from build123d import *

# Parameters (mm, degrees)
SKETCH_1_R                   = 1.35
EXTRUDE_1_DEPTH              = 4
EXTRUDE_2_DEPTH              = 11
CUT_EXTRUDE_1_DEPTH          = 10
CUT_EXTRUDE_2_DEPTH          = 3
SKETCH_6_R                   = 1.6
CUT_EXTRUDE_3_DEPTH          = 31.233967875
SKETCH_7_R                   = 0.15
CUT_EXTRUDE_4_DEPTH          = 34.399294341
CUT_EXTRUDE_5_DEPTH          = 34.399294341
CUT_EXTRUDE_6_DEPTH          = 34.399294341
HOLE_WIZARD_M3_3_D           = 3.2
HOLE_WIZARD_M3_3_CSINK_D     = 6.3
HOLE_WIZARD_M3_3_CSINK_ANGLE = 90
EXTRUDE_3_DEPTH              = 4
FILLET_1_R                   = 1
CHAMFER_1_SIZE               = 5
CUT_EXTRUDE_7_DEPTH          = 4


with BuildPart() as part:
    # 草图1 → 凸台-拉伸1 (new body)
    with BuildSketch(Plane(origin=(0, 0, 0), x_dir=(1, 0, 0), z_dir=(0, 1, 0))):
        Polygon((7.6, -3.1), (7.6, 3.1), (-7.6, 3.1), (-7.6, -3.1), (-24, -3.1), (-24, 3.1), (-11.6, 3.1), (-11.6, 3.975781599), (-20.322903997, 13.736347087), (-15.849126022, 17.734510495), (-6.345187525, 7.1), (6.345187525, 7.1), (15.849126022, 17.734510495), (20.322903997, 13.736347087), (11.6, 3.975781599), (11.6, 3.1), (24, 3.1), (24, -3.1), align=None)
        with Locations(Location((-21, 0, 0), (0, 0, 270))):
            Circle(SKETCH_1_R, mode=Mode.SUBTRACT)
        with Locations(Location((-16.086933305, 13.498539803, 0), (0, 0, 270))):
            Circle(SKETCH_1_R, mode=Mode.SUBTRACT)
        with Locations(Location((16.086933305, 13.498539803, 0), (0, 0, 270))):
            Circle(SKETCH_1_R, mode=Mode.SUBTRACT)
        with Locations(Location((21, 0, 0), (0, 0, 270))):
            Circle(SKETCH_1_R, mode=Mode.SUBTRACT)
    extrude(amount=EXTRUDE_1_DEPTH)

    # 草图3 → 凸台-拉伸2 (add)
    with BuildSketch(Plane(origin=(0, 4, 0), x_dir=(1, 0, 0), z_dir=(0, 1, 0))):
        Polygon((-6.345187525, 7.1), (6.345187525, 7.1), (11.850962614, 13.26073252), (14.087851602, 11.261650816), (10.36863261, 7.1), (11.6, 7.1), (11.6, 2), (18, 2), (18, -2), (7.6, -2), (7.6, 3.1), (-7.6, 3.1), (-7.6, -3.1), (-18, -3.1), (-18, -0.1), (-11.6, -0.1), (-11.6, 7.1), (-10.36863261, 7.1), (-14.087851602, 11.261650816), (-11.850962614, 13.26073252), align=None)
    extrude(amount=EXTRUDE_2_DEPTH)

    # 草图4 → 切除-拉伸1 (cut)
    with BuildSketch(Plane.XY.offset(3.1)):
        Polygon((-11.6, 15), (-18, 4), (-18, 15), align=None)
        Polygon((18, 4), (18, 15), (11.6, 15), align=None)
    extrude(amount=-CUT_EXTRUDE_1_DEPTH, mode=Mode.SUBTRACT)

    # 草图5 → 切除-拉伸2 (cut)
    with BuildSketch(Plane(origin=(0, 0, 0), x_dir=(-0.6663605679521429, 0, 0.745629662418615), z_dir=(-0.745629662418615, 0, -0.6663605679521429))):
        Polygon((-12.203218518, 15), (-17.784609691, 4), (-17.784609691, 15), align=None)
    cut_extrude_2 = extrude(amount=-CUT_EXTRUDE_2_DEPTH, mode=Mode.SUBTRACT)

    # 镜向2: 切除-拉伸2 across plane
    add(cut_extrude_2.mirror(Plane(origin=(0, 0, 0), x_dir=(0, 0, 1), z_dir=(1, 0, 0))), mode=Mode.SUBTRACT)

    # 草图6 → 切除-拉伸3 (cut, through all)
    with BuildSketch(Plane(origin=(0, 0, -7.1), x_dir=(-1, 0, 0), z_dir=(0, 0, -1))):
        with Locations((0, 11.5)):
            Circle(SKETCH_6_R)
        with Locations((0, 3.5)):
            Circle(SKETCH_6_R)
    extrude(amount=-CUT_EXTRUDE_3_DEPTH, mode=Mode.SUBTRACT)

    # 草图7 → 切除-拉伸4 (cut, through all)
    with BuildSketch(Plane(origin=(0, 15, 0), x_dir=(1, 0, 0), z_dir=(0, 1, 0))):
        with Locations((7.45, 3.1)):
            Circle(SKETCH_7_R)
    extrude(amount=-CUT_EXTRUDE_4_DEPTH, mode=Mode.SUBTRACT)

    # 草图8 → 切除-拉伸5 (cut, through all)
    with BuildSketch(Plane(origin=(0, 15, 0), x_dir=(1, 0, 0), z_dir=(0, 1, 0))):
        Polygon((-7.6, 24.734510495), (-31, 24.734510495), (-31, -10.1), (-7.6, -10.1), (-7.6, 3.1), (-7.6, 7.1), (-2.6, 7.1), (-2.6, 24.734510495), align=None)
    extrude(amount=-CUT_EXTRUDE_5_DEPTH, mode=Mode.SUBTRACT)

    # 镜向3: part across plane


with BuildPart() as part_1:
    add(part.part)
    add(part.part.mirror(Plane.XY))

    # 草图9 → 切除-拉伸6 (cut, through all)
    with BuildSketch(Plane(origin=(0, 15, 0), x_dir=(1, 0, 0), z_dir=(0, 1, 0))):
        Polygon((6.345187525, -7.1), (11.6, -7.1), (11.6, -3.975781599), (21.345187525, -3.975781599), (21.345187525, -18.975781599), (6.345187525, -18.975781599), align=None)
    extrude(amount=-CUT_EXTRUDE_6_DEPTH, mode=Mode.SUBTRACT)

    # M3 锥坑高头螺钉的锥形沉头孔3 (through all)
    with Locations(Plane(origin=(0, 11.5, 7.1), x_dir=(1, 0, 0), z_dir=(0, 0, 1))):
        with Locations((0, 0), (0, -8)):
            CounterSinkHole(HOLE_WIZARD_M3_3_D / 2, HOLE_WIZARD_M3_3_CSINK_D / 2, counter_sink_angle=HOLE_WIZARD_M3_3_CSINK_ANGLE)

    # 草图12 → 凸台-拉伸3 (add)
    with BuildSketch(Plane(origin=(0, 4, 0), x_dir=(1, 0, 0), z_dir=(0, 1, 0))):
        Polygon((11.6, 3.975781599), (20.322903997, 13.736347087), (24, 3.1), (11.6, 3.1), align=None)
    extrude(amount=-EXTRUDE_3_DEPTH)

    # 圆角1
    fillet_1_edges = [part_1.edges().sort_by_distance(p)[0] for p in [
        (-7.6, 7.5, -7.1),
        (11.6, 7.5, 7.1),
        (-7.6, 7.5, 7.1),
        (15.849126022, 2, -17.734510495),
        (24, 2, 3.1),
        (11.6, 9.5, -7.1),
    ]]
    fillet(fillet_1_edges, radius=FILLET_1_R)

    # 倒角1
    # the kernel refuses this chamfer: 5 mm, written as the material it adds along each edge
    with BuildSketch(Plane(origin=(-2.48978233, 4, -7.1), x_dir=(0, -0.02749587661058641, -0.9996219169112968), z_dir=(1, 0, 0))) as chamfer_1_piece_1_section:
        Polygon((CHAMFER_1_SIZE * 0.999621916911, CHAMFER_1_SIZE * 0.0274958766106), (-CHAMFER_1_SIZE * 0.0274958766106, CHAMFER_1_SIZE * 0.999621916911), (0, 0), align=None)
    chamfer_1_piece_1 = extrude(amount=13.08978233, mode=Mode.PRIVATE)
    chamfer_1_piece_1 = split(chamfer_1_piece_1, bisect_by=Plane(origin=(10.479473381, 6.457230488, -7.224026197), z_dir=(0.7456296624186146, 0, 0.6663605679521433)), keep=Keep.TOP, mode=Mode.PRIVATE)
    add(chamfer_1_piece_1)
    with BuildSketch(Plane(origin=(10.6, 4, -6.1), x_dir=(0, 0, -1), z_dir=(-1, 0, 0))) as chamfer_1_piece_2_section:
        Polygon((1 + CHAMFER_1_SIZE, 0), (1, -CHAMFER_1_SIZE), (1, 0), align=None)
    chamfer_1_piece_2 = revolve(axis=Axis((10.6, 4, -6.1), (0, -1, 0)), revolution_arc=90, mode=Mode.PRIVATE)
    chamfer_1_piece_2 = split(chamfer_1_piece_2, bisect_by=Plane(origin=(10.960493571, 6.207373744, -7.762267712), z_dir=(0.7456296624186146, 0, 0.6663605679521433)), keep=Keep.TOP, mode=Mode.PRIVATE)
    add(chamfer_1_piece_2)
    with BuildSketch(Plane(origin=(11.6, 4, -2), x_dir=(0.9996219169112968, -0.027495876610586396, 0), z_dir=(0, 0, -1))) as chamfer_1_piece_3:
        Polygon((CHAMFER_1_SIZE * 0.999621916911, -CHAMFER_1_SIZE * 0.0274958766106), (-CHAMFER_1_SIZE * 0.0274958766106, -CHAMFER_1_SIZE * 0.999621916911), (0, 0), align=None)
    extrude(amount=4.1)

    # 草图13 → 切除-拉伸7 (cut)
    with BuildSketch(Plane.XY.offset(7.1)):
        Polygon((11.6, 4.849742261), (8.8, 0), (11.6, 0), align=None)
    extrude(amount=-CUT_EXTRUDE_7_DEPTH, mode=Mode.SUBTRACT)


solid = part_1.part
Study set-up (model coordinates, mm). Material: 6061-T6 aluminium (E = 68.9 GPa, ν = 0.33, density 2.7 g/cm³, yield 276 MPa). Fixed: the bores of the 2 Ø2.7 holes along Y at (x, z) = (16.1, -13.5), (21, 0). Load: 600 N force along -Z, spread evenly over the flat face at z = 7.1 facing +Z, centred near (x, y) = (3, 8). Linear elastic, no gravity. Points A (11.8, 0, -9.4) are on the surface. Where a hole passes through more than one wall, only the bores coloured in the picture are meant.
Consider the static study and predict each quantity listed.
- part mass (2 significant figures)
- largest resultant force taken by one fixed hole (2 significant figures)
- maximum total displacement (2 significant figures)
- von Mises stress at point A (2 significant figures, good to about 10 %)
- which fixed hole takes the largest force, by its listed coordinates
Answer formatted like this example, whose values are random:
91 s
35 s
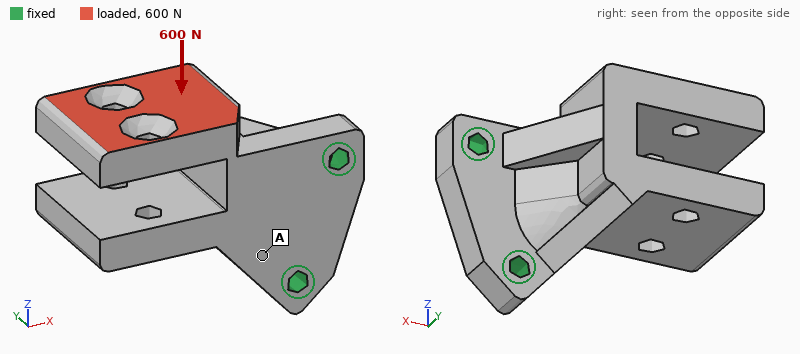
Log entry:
9.9 g
850 N
0.16 mm
13 MPa
(16.1, -13.5)
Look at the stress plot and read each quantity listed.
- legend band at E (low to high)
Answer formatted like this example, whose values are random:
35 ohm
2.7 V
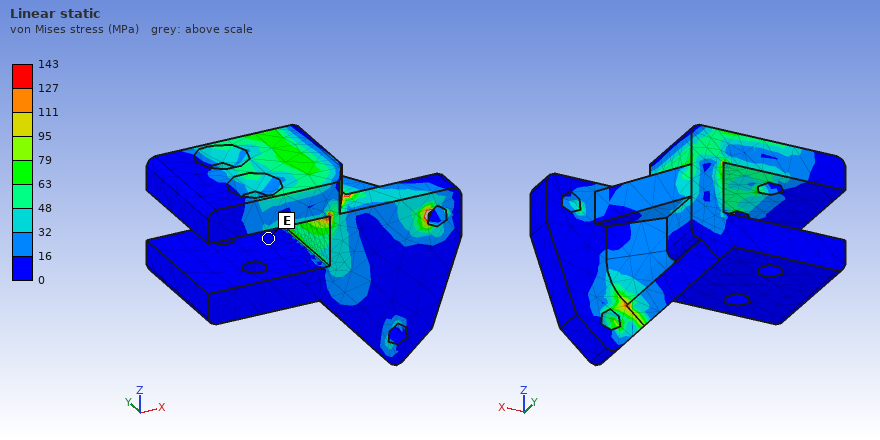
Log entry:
0 to 16 MPa
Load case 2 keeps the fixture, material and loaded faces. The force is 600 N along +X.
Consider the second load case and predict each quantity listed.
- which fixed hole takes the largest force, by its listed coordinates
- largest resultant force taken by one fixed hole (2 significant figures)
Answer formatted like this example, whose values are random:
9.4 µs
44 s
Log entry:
(21, 0)
860 N
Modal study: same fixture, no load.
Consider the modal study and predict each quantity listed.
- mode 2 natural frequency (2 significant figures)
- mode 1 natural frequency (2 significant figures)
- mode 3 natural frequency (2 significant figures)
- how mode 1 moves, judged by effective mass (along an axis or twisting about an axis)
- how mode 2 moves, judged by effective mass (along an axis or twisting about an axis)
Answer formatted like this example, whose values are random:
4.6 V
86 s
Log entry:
6800 Hz
3800 Hz
10 kHz
along Y
along Z
